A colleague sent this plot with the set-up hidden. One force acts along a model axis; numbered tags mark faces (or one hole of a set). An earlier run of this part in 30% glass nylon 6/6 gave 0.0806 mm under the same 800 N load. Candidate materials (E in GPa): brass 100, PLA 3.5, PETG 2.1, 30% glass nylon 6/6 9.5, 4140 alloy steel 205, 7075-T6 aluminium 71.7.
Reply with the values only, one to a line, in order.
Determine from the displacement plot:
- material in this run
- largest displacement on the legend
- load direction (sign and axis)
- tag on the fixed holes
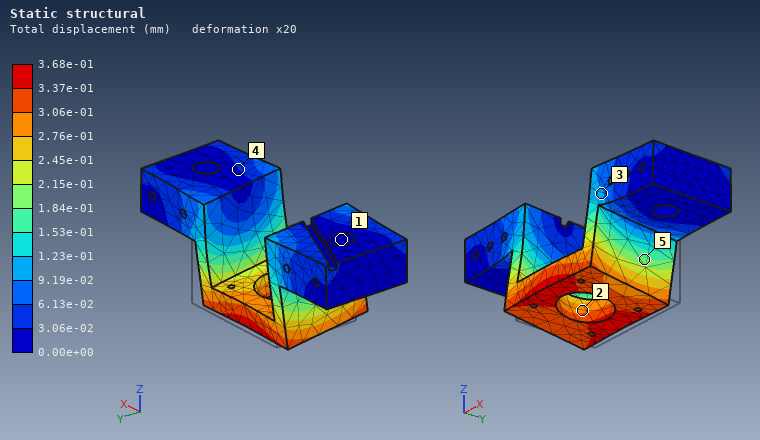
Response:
PETG
3.68e-01 mm
-Y
1
